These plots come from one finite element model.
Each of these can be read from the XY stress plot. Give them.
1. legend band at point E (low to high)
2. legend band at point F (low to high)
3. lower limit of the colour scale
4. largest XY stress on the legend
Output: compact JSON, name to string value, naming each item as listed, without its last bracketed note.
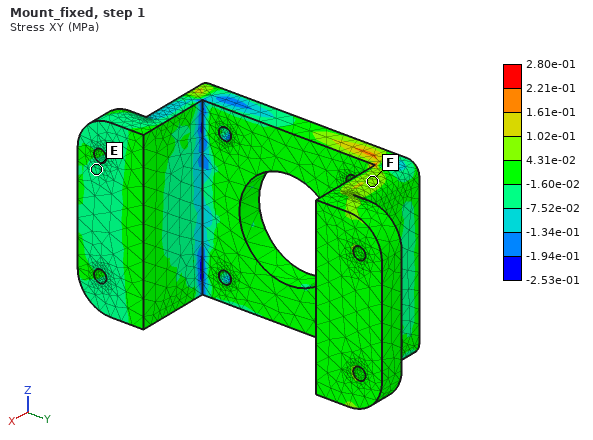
{"legend band at point E": "-7.52e-02 to -1.60e-02 MPa", "legend band at point F": "4.31e-02 to 1.02e-01 MPa", "lower limit of the colour scale": "-2.53e-01 MPa", "largest XY stress on the legend": "2.80e-01 MPa"}
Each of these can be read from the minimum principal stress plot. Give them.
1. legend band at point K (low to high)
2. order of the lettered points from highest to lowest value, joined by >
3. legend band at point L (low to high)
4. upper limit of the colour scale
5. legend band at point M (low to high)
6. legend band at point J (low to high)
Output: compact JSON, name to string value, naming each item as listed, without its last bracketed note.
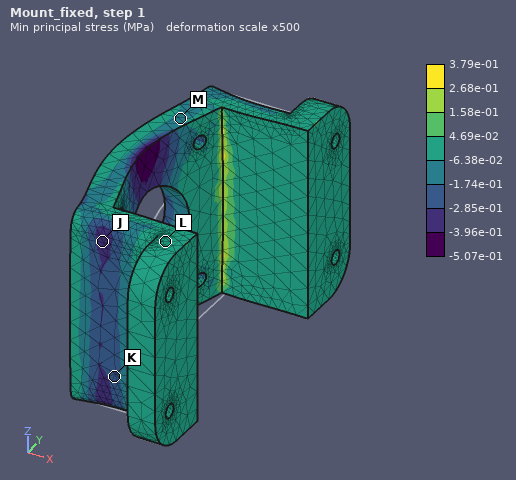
{"legend band at point K": "-2.85e-01 to -1.74e-01 MPa", "order of the lettered points from highest to lowest value, joined by >": "L > M > K > J", "legend band at point L": "-6.38e-02 to 4.69e-02 MPa", "upper limit of the colour scale": "3.79e-01 MPa", "legend band at point M": "-1.74e-01 to -6.38e-02 MPa", "legend band at point J": "-3.96e-01 to -2.85e-01 MPa"}
